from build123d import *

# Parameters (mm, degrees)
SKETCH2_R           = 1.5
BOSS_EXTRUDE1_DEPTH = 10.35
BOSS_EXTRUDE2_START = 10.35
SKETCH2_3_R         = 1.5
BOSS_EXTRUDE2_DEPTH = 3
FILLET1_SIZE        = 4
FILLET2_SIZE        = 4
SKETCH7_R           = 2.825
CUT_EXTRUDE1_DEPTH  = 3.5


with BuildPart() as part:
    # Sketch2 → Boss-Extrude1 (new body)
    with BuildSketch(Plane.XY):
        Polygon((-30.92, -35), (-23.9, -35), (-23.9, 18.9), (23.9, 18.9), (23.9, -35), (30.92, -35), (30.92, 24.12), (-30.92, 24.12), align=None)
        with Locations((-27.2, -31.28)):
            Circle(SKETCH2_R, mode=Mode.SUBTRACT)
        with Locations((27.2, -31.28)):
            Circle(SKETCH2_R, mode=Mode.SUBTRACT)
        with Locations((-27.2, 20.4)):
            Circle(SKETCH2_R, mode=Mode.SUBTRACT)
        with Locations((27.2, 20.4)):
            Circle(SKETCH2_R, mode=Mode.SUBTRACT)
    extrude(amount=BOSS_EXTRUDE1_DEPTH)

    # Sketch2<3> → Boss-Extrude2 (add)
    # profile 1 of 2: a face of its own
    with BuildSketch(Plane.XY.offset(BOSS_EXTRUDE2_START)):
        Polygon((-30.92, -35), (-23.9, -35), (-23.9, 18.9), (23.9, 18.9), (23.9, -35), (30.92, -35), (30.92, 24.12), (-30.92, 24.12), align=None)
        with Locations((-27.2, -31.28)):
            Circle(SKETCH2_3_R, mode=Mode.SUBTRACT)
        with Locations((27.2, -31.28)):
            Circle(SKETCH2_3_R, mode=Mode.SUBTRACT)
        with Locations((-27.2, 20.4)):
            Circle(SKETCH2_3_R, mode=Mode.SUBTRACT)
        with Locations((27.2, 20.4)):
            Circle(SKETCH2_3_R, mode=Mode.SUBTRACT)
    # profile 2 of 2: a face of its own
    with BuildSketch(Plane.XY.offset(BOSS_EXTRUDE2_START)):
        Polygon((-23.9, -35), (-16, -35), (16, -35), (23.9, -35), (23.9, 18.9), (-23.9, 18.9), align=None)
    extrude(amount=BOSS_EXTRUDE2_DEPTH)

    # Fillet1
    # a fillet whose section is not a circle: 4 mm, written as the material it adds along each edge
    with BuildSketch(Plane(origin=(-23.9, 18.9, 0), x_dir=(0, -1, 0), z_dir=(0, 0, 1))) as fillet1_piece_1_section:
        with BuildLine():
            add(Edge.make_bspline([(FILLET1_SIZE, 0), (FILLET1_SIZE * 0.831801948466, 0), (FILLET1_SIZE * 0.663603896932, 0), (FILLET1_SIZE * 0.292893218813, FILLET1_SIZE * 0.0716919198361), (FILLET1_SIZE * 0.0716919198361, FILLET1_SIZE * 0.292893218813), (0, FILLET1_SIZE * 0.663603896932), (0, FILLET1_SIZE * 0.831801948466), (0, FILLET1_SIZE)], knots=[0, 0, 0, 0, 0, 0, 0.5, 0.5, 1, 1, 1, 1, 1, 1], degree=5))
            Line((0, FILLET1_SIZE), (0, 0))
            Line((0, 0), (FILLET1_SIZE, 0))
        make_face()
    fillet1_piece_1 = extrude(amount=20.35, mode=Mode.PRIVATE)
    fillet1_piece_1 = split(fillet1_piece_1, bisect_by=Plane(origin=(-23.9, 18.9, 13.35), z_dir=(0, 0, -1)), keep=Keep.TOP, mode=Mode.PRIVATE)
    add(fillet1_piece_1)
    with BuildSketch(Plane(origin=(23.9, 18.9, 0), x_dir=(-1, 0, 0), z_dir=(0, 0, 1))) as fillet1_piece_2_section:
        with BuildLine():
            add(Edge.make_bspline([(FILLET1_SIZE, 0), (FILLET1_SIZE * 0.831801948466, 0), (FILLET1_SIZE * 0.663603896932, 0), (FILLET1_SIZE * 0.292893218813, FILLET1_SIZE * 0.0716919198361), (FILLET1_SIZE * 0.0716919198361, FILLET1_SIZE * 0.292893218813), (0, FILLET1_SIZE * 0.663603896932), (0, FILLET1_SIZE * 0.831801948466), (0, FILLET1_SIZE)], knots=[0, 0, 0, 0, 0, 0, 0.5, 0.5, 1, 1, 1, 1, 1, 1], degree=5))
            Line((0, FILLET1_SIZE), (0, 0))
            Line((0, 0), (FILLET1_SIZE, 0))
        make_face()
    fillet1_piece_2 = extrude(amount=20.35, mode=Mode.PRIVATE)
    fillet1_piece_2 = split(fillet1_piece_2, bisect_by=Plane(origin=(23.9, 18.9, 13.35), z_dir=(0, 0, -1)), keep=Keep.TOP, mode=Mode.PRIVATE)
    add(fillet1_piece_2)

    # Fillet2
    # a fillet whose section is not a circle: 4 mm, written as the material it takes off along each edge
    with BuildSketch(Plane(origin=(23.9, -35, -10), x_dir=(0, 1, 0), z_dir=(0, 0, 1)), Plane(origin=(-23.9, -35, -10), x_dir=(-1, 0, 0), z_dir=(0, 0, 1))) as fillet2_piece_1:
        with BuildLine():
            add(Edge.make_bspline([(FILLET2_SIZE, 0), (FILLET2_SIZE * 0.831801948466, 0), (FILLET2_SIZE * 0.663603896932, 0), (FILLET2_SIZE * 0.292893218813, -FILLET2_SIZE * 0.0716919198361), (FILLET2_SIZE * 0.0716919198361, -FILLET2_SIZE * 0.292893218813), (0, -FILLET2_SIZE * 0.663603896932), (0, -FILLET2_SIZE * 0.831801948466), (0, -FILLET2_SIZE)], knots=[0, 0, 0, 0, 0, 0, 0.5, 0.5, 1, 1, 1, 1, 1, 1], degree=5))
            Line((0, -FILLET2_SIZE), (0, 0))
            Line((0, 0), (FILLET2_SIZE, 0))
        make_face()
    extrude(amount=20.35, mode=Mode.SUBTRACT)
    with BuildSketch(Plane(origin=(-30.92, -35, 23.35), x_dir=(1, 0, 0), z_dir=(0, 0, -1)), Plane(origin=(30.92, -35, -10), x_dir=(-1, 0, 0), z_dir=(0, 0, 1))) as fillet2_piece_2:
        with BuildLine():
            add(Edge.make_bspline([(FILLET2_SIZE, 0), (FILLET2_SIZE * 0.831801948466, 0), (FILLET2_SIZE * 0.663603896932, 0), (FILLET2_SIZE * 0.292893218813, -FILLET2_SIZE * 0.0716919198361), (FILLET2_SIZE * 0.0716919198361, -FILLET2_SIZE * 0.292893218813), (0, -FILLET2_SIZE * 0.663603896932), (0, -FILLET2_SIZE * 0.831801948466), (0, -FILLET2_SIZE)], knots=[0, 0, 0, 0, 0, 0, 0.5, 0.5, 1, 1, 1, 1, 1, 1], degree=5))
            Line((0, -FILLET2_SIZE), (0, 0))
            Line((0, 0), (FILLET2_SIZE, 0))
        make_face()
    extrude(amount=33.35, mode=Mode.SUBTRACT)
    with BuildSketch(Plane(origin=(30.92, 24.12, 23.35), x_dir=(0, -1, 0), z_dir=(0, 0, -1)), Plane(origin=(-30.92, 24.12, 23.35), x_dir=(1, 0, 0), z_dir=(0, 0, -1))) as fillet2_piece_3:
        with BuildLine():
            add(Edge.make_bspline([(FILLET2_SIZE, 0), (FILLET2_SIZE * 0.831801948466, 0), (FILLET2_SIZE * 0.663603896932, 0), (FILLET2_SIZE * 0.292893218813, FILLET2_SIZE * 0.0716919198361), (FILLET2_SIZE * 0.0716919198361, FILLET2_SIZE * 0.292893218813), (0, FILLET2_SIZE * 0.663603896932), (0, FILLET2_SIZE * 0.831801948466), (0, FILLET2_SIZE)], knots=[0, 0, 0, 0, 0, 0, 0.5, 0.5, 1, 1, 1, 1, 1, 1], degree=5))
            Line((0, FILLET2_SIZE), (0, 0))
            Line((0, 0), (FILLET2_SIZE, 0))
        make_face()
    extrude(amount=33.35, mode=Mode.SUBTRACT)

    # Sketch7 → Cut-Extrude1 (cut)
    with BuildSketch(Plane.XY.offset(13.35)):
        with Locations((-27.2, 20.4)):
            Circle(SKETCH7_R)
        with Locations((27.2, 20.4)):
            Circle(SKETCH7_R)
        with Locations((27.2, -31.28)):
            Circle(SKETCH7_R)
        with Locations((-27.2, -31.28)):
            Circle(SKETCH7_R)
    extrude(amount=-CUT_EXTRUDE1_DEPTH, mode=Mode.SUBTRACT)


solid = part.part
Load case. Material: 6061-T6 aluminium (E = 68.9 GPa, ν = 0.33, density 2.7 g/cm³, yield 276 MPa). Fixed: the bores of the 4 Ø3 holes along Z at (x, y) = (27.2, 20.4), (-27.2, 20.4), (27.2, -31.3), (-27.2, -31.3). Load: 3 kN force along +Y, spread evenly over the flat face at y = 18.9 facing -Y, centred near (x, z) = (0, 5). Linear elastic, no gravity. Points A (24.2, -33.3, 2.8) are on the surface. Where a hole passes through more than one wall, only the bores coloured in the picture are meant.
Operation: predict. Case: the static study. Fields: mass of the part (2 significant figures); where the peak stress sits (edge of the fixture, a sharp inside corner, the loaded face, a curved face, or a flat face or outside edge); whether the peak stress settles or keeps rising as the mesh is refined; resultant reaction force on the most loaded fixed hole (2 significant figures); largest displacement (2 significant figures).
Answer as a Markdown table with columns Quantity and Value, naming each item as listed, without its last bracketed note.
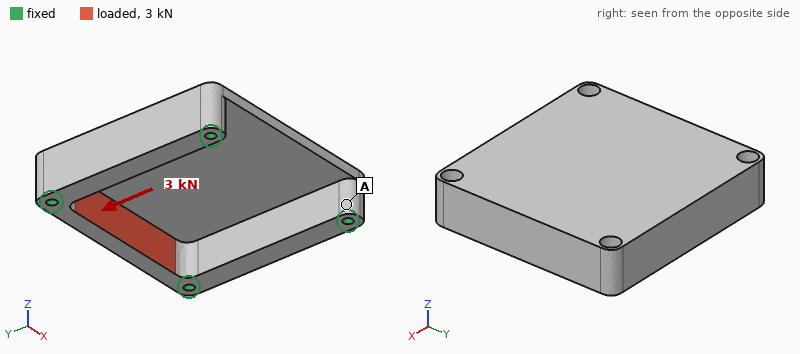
| Quantity | Value |
|---|---|
| mass of the part | 58 g |
| where the peak stress sits | edge of the fixture |
| whether the peak stress settles or keeps rising as the mesh is refined | keeps rising |
| resultant reaction force on the most loaded fixed hole | 1.1 kN |
| largest displacement | 76 µm |
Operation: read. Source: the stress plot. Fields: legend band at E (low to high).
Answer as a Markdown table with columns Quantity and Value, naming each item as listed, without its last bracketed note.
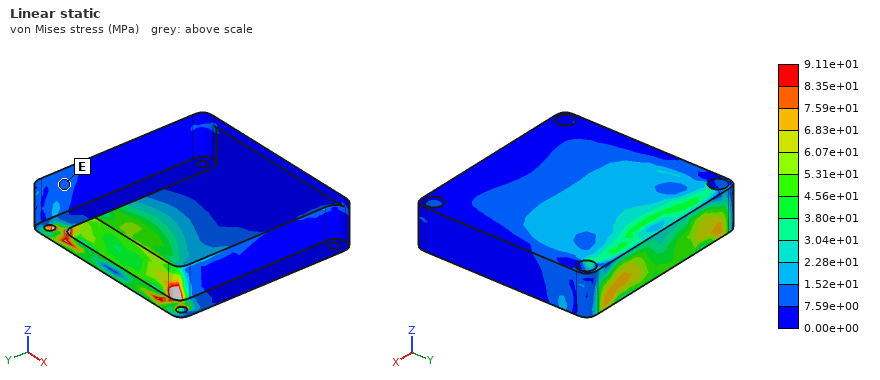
| Quantity | Value |
|---|---|
| legend band at E | 7.59e+00 to 1.52e+01 MPa |
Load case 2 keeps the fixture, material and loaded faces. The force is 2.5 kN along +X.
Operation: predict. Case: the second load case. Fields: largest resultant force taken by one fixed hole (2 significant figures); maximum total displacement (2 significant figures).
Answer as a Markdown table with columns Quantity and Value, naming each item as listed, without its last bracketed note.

| Quantity | Value |
|---|---|
| largest resultant force taken by one fixed hole | 1.2 kN |
| maximum total displacement | 5.8 µm |
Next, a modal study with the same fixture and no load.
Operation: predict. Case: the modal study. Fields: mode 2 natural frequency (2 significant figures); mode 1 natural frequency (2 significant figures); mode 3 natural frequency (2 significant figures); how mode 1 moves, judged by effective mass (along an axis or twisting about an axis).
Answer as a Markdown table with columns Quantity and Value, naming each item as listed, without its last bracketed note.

| Quantity | Value |
|---|---|
| mode 2 natural frequency | 8700 Hz |
| mode 1 natural frequency | 5800 Hz |
| mode 3 natural frequency | 13 kHz |
| how mode 1 moves, judged by effective mass | along Z |
